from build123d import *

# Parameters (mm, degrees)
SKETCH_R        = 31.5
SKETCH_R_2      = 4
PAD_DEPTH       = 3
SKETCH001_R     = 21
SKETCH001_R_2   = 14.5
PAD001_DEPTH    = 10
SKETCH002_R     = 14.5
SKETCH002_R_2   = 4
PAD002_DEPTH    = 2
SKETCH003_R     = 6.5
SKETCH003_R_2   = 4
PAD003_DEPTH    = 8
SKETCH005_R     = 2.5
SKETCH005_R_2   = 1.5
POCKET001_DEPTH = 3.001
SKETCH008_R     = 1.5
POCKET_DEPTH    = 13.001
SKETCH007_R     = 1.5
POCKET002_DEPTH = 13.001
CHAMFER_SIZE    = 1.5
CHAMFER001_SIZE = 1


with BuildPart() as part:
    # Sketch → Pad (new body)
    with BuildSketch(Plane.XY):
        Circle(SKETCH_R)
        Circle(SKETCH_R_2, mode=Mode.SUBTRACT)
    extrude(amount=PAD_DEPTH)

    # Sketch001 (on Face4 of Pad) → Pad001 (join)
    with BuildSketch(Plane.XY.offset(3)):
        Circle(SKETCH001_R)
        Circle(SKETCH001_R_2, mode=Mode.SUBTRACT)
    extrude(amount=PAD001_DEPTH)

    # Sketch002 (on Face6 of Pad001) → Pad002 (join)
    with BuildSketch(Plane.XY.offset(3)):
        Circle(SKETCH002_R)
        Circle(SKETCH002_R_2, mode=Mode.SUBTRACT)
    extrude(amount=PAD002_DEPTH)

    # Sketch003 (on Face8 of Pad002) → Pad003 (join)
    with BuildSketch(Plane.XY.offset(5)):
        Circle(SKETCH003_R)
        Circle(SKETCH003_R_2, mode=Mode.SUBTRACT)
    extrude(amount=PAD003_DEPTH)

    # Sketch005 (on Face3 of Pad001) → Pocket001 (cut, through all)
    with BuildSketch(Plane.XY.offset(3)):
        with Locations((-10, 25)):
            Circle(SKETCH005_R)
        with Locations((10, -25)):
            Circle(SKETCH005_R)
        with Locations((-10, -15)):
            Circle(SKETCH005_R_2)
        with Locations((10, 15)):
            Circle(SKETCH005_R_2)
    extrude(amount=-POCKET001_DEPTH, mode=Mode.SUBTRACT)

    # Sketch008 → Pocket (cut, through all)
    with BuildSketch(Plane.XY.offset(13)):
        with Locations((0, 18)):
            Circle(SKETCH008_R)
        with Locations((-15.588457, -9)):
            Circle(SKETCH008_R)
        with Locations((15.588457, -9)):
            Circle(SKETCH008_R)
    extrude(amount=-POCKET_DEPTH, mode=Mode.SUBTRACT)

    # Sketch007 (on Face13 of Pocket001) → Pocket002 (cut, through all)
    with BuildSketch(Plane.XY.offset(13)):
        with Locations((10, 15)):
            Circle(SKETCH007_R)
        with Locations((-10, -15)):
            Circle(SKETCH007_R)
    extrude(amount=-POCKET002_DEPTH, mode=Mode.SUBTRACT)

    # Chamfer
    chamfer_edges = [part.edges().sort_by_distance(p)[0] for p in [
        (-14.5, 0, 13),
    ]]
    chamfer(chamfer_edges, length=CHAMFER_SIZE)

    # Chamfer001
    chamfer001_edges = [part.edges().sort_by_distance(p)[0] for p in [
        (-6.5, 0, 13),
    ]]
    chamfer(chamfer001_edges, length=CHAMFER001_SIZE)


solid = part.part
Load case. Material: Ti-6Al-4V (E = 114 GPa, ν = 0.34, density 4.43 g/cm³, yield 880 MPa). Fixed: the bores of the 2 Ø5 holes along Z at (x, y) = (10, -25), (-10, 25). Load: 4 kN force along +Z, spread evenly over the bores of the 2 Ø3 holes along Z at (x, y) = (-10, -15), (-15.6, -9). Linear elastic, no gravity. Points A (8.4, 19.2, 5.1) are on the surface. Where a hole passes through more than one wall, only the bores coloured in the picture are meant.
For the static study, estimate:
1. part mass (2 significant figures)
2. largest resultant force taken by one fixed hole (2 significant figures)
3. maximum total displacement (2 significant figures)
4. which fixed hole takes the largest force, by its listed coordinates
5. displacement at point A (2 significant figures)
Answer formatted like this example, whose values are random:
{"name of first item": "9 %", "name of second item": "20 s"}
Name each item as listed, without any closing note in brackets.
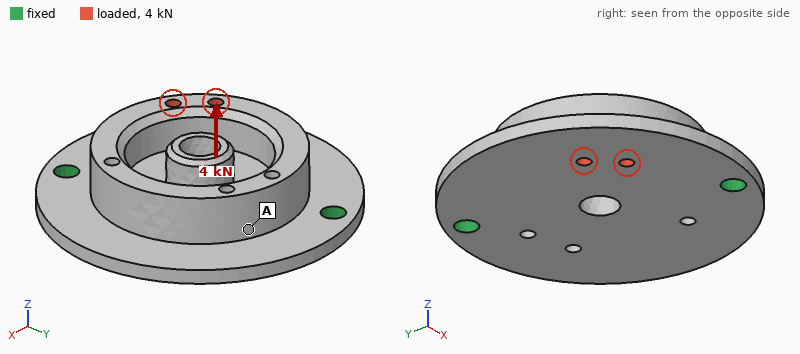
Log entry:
{"part mass": "78 g", "largest resultant force taken by one fixed hole": "3.1 kN", "maximum total displacement": "0.68 mm", "which fixed hole takes the largest force, by its listed coordinates": "(10, -25)", "displacement at point A": "0.22 mm"}
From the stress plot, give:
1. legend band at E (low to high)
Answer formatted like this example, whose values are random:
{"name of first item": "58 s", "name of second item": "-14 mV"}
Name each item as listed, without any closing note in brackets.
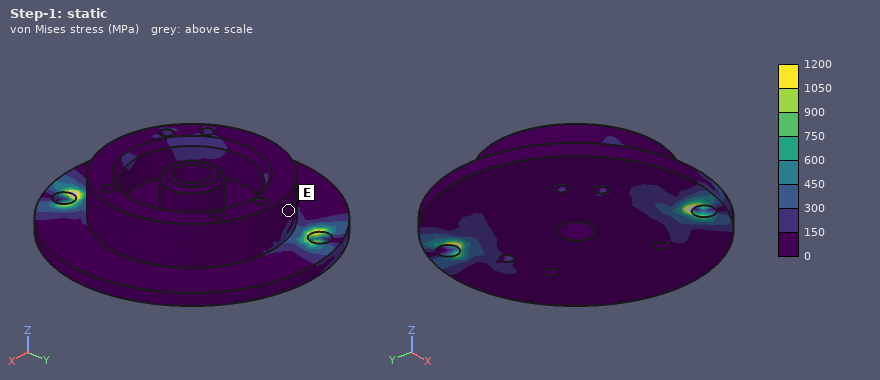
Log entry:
{"legend band at E": "0 to 150 MPa"}
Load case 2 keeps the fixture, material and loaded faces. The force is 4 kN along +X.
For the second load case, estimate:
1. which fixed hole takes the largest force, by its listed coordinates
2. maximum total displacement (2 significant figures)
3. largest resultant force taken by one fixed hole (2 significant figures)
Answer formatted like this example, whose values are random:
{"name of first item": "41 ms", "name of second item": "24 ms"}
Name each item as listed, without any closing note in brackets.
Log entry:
{"which fixed hole takes the largest force, by its listed coordinates": "(10, -25)", "maximum total displacement": "0.18 mm", "largest resultant force taken by one fixed hole": "2.9 kN"}
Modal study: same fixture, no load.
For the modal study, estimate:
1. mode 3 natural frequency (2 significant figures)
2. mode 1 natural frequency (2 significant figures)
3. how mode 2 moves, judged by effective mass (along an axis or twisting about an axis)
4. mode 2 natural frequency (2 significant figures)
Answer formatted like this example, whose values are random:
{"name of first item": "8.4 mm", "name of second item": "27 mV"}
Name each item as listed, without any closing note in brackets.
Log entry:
{"mode 3 natural frequency": "11 kHz", "mode 1 natural frequency": "2300 Hz", "how mode 2 moves, judged by effective mass": "along Z", "mode 2 natural frequency": "5300 Hz"}
